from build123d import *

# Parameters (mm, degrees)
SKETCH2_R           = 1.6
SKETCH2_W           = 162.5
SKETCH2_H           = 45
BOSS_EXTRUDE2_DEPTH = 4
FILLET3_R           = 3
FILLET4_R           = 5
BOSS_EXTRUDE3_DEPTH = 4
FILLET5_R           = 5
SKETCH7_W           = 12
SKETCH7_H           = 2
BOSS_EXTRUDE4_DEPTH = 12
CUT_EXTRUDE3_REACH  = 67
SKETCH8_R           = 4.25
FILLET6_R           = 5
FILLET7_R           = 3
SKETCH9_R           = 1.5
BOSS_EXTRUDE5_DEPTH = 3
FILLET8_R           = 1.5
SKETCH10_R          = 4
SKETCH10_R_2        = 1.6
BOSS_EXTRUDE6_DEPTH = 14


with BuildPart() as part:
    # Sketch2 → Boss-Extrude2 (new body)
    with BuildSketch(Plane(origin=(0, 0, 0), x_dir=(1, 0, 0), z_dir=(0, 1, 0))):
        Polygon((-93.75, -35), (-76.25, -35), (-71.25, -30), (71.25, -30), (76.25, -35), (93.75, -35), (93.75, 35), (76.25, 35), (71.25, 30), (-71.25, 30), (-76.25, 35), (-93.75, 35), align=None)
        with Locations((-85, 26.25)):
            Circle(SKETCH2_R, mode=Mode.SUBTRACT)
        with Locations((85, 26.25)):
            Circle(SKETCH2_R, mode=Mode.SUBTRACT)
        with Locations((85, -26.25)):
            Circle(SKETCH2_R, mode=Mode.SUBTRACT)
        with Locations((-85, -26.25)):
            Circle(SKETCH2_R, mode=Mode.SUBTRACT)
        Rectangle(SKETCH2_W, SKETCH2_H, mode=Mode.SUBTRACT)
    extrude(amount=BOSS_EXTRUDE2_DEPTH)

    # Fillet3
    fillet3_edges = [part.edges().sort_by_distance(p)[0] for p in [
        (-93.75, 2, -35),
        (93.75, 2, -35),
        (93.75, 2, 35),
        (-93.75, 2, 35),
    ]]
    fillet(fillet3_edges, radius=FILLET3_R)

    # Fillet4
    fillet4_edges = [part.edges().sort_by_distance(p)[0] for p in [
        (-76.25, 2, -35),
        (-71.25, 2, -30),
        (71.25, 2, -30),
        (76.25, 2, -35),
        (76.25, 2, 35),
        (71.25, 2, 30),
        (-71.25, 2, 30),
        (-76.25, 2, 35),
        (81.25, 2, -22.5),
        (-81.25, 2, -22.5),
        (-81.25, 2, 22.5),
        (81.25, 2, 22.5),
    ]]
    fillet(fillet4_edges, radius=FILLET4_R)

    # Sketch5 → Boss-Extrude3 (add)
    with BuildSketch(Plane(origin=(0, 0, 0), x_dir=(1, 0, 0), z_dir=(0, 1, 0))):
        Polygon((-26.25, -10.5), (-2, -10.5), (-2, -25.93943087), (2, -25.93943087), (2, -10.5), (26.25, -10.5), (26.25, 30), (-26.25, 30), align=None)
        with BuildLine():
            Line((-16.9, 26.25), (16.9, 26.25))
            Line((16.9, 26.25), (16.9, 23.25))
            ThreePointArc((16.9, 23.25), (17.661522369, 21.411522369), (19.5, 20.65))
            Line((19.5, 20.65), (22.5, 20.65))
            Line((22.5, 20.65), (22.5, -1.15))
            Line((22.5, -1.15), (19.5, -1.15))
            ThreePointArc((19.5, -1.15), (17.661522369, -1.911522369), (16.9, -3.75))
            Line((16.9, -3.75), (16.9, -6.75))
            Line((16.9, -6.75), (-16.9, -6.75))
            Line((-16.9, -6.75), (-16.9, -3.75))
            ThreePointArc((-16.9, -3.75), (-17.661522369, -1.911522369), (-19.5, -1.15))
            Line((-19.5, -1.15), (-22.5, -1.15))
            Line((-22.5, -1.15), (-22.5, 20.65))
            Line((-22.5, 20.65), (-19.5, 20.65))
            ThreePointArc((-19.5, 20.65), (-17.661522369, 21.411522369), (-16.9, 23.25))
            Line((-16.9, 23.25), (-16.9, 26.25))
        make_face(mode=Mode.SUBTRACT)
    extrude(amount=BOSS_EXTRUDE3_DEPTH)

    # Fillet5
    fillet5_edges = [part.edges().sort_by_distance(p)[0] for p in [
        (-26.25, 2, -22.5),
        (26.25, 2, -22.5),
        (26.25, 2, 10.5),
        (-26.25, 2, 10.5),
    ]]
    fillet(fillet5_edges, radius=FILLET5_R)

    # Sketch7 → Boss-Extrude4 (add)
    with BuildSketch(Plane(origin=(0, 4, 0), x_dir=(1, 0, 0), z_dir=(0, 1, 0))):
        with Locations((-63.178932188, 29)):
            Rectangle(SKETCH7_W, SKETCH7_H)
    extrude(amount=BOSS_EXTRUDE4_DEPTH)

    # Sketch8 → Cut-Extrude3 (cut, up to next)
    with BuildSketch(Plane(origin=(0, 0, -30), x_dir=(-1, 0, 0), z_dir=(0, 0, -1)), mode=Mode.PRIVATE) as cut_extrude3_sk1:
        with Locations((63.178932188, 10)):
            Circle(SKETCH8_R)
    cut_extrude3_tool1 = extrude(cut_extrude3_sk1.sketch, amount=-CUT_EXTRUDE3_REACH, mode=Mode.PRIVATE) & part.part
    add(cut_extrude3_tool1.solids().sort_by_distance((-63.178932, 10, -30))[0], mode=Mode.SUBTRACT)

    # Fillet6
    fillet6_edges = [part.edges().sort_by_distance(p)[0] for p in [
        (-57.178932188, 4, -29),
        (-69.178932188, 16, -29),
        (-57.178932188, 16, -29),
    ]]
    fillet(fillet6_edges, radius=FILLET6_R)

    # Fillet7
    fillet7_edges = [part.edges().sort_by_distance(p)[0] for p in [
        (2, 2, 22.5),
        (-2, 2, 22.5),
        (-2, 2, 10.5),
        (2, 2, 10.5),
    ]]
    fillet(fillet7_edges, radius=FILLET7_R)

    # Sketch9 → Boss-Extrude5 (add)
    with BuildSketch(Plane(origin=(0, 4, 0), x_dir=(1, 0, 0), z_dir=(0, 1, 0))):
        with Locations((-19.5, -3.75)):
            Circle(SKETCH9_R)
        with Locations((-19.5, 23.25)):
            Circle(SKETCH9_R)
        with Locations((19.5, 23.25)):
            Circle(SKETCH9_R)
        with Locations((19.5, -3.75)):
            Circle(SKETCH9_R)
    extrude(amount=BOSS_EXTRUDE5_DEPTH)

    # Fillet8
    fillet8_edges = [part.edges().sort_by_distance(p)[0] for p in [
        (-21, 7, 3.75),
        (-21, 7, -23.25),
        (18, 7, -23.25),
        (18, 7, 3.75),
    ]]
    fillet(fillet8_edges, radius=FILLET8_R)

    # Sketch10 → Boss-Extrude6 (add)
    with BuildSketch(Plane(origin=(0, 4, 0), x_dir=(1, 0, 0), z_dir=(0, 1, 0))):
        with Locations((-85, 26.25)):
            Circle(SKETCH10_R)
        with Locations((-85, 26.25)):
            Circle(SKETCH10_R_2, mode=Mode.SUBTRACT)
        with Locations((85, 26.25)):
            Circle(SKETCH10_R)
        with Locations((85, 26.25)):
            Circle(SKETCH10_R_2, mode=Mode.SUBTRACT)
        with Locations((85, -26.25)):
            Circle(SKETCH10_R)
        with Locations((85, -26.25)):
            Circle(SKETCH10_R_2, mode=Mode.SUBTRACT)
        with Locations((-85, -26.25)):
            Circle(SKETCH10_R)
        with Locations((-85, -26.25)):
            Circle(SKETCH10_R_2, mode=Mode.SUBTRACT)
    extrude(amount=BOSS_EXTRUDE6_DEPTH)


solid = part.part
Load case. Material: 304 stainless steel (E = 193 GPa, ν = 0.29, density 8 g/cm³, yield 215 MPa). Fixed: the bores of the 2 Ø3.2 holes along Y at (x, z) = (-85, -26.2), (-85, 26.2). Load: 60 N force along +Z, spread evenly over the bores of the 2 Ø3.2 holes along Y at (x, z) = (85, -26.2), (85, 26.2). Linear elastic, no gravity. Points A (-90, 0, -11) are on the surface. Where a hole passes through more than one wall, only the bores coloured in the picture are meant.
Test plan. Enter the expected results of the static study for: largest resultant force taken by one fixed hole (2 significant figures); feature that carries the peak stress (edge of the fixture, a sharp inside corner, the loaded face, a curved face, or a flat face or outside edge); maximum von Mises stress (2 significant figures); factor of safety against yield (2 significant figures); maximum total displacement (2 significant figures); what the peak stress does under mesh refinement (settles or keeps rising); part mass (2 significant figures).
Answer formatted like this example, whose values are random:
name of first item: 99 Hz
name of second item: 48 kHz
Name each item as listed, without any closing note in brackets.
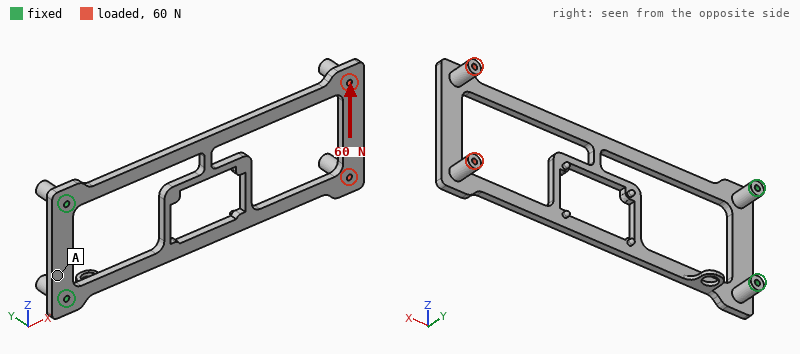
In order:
largest resultant force taken by one fixed hole: 170 N
feature that carries the peak stress: a curved face
maximum von Mises stress: 62 MPa
factor of safety against yield: 3.5
maximum total displacement: 0.18 mm
what the peak stress does under mesh refinement: settles
part mass: 180 g
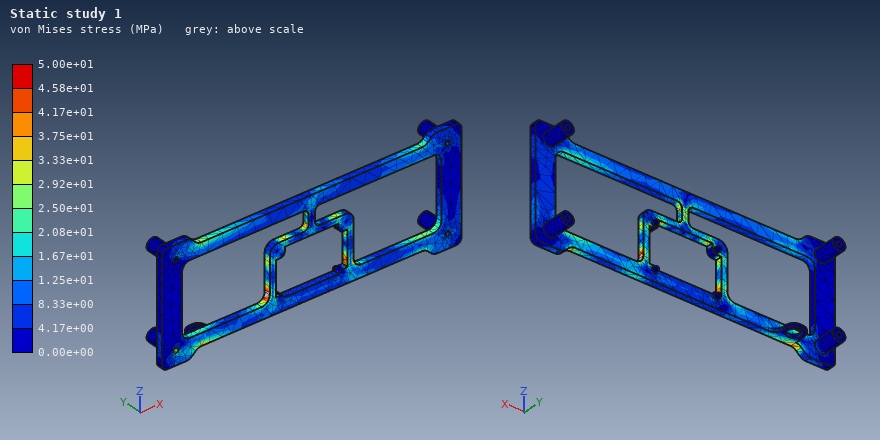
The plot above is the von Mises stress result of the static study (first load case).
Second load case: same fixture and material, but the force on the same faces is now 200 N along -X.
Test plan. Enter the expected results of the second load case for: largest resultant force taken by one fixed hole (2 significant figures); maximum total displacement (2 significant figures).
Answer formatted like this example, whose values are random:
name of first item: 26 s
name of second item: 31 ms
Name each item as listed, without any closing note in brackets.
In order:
largest resultant force taken by one fixed hole: 100 N
maximum total displacement: 1.3 mm
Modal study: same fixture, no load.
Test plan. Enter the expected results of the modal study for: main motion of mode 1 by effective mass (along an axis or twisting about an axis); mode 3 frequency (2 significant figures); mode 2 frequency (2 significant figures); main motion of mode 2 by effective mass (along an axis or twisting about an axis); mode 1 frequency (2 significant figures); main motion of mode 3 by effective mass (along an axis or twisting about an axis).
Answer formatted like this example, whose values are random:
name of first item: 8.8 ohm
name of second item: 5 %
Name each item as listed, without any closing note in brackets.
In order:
main motion of mode 1 by effective mass: along Y
mode 3 frequency: 450 Hz
mode 2 frequency: 300 Hz
main motion of mode 2 by effective mass: twisting about X
mode 1 frequency: 69 Hz
main motion of mode 3 by effective mass: along Z
